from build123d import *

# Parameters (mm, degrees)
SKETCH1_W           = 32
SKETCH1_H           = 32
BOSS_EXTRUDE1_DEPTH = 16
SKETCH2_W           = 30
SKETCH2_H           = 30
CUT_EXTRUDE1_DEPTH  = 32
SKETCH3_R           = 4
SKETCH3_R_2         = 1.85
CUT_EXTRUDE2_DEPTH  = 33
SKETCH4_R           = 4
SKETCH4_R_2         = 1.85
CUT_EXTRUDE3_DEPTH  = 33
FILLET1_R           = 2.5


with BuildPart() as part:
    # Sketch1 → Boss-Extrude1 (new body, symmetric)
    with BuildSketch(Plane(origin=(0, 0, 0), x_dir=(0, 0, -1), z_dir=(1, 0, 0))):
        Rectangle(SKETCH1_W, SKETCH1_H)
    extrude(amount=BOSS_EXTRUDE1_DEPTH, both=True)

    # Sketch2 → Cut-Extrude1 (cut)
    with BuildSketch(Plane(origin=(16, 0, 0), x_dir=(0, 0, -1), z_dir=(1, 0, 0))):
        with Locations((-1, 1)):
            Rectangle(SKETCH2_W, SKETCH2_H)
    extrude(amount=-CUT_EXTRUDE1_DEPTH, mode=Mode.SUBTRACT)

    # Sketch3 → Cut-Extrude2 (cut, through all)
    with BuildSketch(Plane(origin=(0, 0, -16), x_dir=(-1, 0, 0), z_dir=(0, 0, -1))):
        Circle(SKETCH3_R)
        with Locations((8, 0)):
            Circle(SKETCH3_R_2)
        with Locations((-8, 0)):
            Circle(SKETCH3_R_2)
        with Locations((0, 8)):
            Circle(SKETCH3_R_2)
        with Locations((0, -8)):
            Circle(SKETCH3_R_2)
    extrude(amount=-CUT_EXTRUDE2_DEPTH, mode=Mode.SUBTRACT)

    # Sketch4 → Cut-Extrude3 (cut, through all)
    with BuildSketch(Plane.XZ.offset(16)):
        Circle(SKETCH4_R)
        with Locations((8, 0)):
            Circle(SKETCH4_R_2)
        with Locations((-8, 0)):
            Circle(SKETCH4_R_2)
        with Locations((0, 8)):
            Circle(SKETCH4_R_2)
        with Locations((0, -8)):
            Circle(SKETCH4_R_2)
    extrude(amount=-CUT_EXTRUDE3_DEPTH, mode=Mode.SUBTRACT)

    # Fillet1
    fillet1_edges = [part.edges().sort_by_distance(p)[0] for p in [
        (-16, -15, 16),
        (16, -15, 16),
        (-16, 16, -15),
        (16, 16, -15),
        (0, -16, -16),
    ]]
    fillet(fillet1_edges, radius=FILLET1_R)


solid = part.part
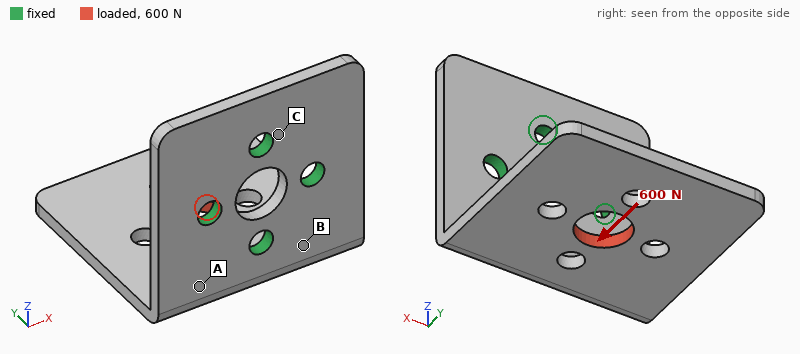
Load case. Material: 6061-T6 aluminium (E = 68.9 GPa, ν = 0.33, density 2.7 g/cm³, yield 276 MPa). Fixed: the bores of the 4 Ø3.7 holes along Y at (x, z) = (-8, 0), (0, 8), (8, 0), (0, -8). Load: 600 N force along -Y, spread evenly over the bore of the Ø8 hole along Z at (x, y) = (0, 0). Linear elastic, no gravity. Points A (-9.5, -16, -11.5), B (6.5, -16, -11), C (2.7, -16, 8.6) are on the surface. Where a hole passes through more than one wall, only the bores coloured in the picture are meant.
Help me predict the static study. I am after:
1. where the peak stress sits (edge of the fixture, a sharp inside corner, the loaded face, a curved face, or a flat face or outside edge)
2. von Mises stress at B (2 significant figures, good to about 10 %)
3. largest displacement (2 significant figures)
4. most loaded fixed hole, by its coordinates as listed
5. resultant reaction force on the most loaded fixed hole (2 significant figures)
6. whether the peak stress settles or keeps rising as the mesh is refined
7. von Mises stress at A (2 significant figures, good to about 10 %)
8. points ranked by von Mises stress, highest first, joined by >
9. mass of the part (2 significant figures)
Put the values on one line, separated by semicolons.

edge of the fixture; 82 MPa; 0.34 mm; (0, -8); 690 N; keeps rising; 55 MPa; B > A > C; 9.6 g
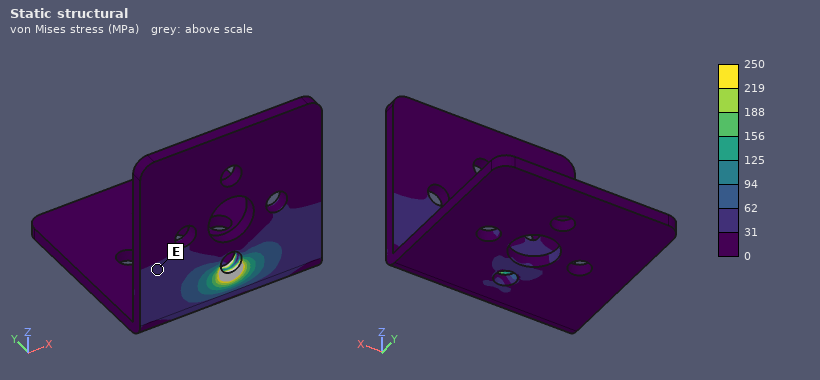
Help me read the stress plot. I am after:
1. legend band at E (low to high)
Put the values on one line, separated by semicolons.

31 to 62 MPa
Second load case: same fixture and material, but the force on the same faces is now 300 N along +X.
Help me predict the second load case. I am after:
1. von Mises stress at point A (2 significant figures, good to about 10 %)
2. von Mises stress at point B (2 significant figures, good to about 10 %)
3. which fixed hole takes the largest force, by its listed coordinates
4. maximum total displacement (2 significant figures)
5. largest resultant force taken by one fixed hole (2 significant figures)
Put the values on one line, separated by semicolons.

46 MPa; 54 MPa; (0, -8); 0.35 mm; 270 N
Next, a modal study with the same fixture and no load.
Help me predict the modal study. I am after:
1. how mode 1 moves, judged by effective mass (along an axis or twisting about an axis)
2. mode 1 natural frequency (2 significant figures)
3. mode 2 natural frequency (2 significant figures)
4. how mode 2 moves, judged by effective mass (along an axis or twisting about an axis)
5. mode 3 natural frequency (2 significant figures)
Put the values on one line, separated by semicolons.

along Z; 1300 Hz; 2300 Hz; along X; 3600 Hz
